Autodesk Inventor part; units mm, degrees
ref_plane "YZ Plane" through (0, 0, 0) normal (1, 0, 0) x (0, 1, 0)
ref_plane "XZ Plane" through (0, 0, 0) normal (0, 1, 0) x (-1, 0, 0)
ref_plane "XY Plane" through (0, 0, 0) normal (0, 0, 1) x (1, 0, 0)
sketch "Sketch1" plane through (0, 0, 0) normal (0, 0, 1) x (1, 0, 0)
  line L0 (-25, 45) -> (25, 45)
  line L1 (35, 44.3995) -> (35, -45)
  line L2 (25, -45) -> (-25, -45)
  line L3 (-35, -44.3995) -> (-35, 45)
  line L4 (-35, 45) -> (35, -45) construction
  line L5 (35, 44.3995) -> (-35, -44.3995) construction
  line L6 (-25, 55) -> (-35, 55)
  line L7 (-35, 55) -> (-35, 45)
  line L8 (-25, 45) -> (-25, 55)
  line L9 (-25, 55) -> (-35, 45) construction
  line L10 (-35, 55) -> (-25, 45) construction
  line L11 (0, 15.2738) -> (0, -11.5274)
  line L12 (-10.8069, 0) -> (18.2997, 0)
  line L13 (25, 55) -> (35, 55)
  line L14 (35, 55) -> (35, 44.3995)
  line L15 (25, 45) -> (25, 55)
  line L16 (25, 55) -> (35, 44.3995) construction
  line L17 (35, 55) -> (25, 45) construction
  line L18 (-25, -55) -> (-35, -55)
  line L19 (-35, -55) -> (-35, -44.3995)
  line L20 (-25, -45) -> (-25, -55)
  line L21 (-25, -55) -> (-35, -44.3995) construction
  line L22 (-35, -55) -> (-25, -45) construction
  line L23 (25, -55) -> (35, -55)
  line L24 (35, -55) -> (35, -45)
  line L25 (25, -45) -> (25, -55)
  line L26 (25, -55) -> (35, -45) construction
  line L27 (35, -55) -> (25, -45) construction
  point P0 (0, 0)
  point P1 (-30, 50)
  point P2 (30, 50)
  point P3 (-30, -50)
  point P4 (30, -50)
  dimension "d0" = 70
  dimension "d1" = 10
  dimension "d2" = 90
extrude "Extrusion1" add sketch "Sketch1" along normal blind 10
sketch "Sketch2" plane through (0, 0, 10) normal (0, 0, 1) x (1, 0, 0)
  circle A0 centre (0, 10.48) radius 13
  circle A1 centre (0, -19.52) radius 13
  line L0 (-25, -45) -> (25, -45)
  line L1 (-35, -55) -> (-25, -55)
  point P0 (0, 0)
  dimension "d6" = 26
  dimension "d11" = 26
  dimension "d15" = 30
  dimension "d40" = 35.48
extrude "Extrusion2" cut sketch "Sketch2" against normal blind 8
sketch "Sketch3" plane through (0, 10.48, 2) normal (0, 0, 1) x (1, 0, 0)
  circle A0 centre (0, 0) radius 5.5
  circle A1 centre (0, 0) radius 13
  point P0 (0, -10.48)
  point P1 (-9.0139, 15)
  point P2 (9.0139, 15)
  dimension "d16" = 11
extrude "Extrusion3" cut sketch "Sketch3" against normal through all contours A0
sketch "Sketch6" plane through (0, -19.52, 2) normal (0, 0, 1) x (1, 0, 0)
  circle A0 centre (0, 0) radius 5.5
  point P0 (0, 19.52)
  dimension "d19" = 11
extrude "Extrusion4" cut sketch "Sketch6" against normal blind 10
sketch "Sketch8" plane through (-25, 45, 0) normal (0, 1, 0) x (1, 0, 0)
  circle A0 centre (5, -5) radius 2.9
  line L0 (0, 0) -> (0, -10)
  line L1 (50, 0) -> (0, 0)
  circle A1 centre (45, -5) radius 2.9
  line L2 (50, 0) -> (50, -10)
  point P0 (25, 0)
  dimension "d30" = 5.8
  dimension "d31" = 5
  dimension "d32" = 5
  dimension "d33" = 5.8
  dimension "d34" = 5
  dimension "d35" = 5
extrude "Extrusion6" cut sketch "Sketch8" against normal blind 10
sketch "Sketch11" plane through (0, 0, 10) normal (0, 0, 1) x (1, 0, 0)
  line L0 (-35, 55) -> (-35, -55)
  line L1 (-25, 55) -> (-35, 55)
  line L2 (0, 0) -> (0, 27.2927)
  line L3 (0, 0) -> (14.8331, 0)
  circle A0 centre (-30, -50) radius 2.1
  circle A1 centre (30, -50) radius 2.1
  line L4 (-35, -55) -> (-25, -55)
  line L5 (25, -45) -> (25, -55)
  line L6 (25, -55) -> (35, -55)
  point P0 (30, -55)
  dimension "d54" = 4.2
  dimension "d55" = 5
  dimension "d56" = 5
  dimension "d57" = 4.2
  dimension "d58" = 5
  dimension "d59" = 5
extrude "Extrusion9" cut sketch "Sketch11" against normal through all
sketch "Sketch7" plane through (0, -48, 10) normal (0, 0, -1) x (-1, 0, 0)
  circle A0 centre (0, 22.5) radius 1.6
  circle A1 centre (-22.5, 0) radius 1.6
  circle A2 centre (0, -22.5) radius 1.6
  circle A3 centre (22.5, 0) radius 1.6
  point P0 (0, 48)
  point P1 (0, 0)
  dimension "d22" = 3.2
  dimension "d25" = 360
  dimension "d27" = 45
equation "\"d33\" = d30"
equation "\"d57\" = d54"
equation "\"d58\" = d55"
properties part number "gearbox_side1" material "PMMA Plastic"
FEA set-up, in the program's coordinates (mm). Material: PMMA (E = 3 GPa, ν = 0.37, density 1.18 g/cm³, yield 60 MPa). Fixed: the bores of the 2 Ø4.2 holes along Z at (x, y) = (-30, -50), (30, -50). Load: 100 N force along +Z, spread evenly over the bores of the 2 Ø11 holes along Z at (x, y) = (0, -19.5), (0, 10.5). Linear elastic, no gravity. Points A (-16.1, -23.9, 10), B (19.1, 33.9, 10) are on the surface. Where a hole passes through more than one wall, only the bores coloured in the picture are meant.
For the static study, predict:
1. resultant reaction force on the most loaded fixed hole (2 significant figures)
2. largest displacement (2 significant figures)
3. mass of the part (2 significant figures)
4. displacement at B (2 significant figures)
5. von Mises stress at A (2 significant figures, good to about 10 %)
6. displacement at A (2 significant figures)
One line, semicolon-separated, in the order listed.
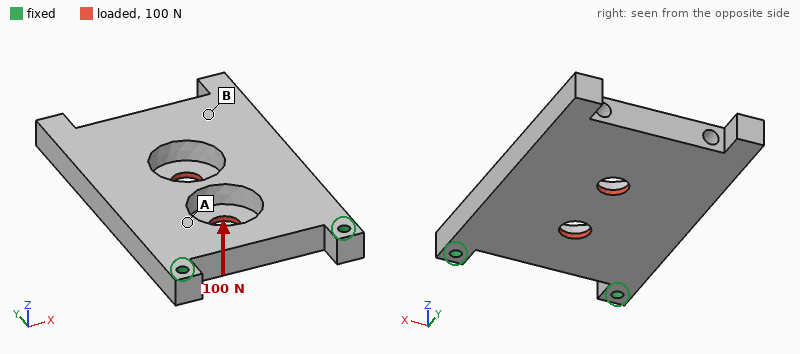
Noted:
50 N; 1.3 mm; 68 g; 1.0 mm; 2.4 MPa; 0.23 mm
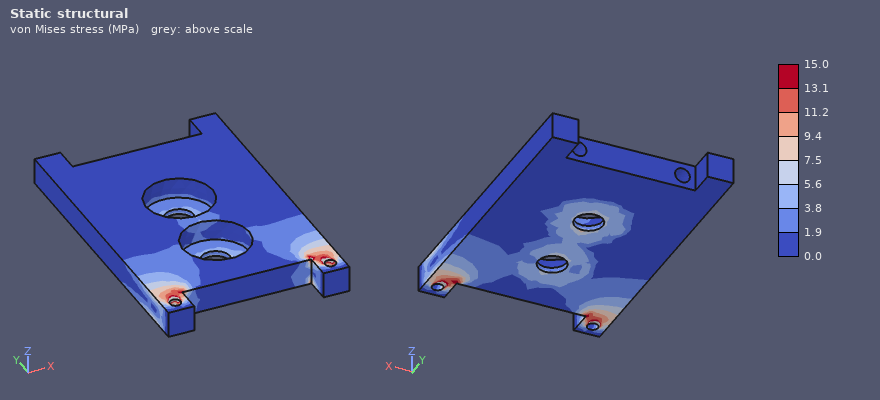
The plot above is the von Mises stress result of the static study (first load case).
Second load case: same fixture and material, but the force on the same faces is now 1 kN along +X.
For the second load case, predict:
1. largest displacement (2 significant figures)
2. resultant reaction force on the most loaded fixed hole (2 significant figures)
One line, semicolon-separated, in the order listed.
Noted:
0.37 mm; 850 N
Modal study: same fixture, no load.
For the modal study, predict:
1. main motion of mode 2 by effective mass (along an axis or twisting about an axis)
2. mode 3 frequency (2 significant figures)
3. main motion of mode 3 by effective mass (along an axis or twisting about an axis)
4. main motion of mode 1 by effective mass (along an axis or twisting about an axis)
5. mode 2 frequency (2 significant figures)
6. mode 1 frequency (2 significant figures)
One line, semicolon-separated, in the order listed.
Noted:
twisting about Y; 1200 Hz; along X; along Z; 650 Hz; 190 Hz
